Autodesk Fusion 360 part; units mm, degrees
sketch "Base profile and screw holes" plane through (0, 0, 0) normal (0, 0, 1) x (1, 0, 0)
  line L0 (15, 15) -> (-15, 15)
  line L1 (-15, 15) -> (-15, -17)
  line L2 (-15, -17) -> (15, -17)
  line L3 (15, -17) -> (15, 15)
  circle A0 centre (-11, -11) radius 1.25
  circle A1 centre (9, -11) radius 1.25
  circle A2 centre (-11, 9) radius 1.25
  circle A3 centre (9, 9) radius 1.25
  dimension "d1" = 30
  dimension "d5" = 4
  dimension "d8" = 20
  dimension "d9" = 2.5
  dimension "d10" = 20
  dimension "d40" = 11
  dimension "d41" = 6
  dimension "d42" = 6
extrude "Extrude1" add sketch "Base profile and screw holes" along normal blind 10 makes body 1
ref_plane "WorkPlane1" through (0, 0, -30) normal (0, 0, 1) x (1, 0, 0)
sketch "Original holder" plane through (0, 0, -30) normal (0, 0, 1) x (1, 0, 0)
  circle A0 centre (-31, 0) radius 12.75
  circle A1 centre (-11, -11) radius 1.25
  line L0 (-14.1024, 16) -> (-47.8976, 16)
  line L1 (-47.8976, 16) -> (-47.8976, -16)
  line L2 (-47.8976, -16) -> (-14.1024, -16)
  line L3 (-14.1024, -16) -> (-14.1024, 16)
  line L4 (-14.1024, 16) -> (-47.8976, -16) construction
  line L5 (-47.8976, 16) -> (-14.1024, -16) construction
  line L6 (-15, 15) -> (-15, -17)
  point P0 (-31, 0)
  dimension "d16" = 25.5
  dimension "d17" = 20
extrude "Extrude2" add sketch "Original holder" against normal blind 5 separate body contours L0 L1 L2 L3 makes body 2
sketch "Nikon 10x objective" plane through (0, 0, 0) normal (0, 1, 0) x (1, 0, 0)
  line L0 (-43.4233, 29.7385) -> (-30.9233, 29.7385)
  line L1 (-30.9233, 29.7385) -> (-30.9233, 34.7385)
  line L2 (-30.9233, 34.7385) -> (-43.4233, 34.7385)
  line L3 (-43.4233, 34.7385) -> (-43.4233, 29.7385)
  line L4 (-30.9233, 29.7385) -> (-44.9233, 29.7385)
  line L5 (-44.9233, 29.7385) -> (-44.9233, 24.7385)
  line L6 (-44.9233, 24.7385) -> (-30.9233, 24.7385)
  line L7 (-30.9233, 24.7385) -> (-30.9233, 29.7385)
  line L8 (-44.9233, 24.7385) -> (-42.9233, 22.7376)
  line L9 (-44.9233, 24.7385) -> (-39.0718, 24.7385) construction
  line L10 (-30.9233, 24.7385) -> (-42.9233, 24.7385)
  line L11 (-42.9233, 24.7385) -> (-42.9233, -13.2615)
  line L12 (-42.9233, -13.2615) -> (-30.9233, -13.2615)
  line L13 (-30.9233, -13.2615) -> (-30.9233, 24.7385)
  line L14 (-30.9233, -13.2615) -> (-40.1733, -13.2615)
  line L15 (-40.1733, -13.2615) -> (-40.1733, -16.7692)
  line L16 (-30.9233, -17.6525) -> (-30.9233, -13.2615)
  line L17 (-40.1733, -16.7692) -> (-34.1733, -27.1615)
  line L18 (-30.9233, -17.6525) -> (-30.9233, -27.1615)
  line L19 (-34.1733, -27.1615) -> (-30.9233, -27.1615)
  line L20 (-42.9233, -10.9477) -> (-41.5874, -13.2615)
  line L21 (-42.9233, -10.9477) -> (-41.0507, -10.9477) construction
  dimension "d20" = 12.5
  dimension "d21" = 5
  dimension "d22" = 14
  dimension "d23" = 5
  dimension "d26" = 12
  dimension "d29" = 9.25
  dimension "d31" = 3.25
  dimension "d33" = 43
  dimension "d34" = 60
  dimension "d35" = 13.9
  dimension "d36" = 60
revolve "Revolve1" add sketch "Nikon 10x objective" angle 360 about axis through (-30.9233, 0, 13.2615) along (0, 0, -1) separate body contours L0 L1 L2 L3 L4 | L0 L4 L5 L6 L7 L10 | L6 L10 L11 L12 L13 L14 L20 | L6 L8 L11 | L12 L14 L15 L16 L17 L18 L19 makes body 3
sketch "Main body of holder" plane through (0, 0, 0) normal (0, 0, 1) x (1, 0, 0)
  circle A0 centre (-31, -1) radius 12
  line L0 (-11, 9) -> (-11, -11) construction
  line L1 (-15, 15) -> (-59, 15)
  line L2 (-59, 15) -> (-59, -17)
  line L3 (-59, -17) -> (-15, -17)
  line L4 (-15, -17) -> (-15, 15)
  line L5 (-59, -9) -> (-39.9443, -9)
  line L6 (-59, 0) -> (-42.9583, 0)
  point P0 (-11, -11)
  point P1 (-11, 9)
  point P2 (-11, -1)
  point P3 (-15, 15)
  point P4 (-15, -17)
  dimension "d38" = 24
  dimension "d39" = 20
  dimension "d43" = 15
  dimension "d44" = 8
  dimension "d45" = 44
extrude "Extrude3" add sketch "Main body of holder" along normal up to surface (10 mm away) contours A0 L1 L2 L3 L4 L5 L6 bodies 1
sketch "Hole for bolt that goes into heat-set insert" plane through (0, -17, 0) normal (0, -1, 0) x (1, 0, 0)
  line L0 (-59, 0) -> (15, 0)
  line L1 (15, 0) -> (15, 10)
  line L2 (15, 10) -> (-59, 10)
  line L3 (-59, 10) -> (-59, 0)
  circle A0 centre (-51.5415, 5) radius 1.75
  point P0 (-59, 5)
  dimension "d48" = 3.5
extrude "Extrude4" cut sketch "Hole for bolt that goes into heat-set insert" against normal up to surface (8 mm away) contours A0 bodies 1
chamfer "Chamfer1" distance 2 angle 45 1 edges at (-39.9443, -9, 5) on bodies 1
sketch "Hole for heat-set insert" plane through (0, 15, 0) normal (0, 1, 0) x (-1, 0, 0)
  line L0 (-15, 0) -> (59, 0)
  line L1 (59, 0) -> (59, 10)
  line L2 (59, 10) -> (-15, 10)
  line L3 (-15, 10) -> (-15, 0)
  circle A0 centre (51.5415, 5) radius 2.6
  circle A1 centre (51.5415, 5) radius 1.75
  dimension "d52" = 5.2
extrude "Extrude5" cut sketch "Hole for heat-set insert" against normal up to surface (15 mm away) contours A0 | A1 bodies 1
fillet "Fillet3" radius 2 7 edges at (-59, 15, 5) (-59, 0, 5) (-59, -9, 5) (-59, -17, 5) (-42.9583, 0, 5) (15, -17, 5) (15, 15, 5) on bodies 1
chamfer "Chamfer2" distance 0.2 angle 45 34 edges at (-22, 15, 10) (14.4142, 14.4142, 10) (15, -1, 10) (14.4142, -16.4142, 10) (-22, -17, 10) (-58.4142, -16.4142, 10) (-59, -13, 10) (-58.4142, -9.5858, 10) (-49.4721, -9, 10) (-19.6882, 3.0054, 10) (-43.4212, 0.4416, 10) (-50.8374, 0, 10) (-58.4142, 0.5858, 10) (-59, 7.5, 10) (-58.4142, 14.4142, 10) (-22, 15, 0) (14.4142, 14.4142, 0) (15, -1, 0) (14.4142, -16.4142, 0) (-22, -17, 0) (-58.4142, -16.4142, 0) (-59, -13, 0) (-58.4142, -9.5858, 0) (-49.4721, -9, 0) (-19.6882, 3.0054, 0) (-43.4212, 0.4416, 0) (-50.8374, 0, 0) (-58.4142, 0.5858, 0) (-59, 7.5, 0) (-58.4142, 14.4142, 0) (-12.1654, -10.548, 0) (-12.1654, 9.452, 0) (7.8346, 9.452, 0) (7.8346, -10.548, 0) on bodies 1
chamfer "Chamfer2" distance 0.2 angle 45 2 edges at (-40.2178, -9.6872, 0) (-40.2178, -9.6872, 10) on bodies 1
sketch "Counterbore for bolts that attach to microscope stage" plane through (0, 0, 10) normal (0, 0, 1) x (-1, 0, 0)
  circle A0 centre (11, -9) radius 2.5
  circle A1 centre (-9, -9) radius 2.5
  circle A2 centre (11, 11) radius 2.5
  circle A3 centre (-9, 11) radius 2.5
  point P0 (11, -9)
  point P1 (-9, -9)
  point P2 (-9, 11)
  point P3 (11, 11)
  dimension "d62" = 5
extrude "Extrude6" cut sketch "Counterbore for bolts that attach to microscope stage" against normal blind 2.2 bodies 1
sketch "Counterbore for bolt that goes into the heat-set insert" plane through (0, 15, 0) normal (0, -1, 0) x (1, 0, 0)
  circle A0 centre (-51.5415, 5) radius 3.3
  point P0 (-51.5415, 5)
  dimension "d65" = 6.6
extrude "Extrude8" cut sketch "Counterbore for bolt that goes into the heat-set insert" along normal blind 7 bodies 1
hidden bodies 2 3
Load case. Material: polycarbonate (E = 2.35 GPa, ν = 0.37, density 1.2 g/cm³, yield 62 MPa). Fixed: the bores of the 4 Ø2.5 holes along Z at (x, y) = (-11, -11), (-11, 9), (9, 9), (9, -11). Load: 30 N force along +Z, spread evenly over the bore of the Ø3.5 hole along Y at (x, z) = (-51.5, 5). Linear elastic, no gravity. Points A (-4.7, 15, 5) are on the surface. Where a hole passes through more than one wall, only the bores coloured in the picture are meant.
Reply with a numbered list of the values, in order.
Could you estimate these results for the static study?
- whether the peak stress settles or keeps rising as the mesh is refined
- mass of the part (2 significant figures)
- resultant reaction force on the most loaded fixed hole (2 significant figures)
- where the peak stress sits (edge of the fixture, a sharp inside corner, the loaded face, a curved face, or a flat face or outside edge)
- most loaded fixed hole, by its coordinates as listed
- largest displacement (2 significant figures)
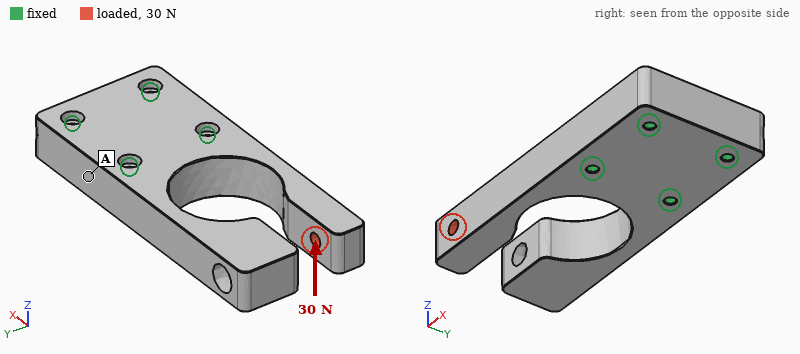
1. keeps rising
2. 20 g
3. 54 N
4. edge of the fixture
5. (-11, -11)
6. 0.74 mm
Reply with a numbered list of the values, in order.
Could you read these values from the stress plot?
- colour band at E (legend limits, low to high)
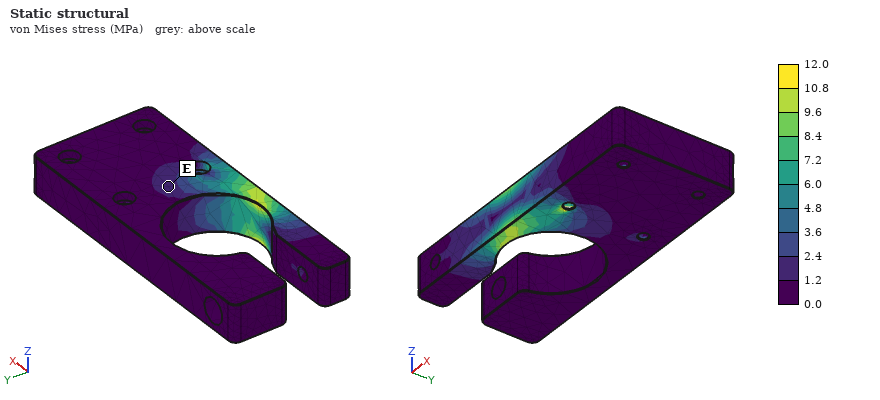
1. 1.2 to 2.4 MPa
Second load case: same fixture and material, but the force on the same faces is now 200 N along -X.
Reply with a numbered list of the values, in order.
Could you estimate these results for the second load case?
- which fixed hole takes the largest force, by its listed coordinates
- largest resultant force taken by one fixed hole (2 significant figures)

1. (-11, -11)
2. 170 N
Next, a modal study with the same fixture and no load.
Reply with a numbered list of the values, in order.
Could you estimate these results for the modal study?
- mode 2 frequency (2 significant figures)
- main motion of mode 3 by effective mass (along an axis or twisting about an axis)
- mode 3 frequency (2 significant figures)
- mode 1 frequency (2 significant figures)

1. 590 Hz
2. along Z
3. 680 Hz
4. 460 Hz
